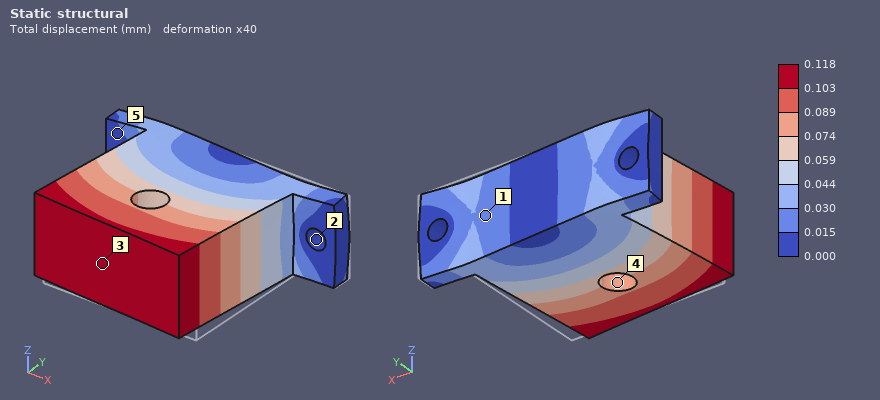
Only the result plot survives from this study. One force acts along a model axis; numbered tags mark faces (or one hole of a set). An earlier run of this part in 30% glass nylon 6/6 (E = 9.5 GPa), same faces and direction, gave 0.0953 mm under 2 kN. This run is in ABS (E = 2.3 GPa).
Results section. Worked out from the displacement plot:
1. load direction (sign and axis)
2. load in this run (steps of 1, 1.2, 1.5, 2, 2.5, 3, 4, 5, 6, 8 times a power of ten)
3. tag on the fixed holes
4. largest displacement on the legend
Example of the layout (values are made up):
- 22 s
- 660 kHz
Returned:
- -X
- 600 N
- 2
- 0.118 mm
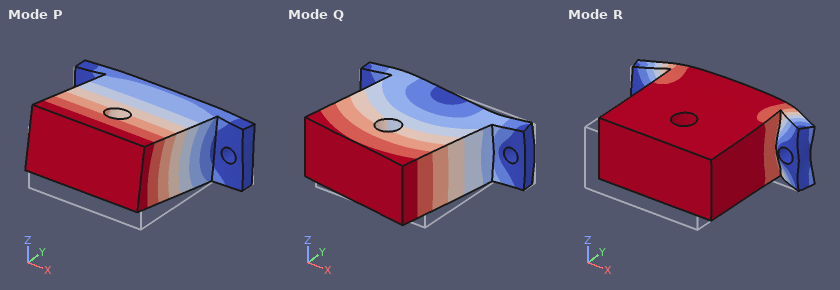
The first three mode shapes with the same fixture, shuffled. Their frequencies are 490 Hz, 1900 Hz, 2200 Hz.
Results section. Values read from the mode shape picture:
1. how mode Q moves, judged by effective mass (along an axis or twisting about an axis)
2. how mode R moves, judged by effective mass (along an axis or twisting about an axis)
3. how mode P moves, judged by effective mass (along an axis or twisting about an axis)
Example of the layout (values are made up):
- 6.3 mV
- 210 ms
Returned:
- along X
- along Y
- along Z
